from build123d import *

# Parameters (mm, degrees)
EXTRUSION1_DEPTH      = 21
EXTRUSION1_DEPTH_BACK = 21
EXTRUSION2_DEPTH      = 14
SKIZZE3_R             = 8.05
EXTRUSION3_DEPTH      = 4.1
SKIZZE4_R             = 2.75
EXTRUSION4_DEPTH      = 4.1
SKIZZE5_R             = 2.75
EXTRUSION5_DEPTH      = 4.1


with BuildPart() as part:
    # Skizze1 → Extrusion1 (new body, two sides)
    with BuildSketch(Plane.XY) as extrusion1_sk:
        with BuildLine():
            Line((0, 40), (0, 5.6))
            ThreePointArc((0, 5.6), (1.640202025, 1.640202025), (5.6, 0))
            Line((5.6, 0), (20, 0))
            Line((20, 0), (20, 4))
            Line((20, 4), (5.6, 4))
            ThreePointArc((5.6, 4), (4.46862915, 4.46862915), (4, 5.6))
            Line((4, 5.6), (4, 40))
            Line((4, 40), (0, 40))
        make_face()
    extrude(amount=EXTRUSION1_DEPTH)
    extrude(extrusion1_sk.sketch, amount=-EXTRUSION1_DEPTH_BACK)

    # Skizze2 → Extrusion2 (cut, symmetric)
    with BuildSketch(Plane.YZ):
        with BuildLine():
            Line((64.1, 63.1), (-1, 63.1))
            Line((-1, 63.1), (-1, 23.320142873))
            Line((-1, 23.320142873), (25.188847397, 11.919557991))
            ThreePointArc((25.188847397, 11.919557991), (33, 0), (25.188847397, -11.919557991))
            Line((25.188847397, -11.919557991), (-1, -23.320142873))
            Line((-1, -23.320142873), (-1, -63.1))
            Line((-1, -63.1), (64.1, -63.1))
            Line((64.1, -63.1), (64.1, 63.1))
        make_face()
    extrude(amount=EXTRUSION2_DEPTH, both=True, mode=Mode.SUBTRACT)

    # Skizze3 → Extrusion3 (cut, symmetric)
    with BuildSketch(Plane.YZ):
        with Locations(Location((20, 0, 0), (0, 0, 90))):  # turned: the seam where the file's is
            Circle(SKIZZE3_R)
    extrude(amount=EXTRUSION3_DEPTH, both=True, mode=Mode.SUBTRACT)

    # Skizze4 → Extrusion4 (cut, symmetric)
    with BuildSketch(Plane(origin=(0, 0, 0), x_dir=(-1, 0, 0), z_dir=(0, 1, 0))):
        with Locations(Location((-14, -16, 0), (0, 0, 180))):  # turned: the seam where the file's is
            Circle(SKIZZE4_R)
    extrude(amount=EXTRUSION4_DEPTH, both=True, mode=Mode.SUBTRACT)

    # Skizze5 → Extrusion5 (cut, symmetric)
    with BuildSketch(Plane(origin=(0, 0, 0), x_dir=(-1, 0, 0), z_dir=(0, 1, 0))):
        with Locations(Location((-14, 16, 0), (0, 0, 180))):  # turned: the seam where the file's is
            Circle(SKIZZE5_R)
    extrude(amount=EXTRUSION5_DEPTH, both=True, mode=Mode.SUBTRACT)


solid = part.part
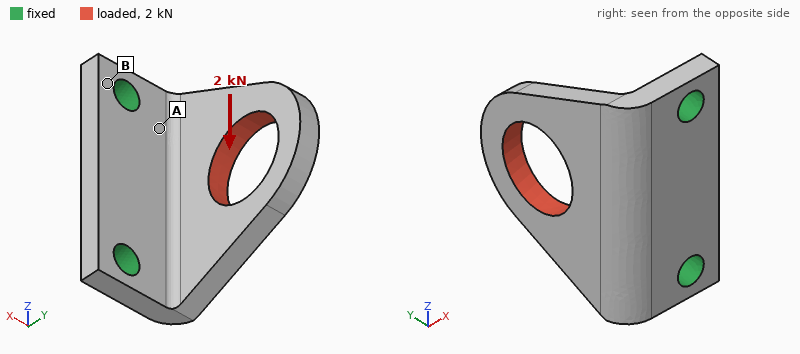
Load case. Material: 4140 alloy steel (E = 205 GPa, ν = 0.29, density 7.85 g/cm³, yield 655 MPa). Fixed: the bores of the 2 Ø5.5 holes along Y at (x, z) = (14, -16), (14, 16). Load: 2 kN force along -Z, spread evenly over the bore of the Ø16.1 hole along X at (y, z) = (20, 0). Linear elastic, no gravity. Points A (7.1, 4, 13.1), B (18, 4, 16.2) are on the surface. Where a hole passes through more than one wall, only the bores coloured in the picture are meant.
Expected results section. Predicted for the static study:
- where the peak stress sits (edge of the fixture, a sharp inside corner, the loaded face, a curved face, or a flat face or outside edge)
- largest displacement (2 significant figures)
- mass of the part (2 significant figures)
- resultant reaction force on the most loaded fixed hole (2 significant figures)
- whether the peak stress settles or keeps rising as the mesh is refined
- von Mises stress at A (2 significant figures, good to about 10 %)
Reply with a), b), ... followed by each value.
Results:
a) edge of the fixture
b) 51 µm
c) 43 g
d) 1.6 kN
e) keeps rising
f) 110 MPa
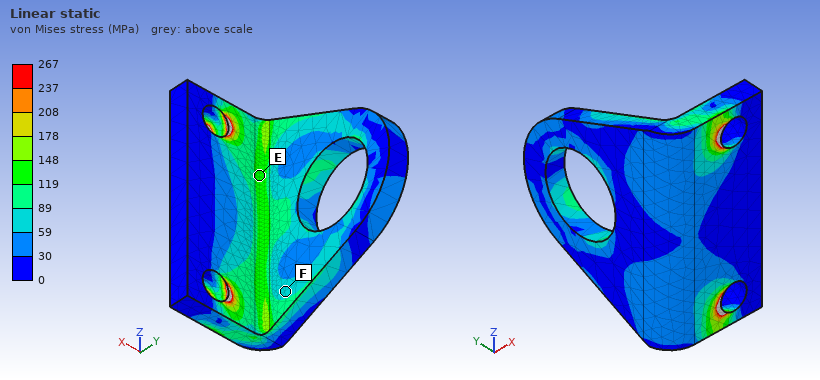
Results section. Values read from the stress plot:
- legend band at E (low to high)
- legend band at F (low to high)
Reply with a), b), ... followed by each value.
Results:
a) 119 to 148 MPa
b) 59 to 89 MPa
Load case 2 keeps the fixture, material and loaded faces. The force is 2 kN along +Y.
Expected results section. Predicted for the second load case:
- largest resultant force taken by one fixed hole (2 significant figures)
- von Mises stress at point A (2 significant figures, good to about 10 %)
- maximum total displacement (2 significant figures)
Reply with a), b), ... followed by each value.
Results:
a) 1.0 kN
b) 99 MPa
c) 100 µm
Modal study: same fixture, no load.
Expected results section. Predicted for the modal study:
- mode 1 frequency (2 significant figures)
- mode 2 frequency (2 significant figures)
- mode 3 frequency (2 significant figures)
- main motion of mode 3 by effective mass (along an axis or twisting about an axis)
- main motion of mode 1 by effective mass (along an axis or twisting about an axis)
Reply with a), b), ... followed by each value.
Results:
a) 3500 Hz
b) 8300 Hz
c) 10 kHz
d) along Y
e) along X
